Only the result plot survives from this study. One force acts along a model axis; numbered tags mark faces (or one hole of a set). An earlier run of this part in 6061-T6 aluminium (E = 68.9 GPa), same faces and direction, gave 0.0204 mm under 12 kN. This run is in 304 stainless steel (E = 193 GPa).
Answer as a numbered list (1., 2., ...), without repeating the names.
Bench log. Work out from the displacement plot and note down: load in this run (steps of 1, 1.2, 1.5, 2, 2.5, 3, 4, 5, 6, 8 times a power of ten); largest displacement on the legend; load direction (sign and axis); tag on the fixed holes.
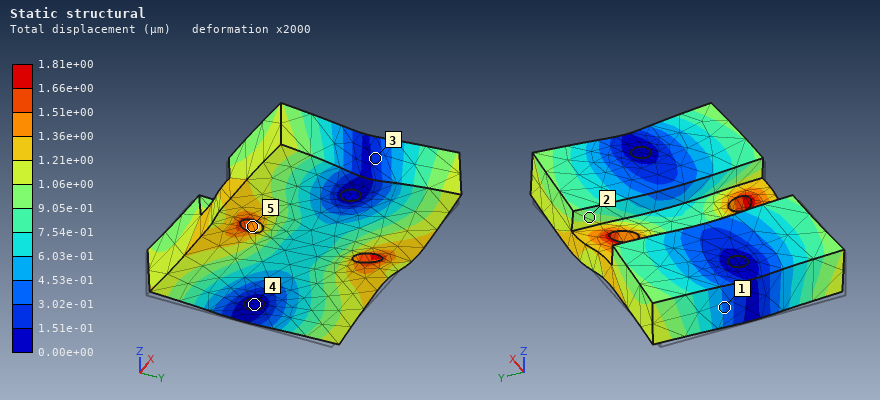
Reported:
1. 3 kN
2. 1.81e+00 µm
3. +X
4. 4
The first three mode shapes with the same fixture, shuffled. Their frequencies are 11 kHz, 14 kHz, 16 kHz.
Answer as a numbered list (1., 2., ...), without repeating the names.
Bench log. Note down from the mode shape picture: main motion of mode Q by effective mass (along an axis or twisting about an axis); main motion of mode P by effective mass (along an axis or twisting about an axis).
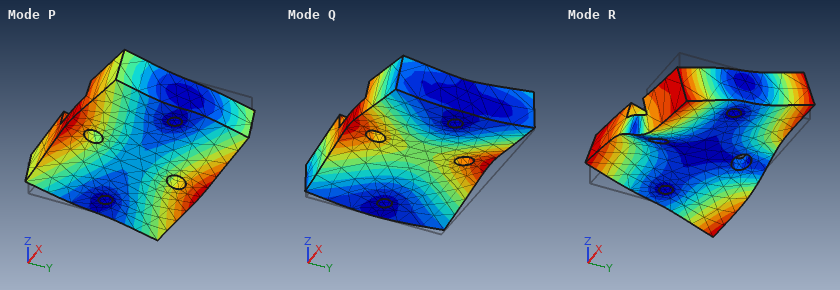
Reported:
1. along Z
2. twisting about X
